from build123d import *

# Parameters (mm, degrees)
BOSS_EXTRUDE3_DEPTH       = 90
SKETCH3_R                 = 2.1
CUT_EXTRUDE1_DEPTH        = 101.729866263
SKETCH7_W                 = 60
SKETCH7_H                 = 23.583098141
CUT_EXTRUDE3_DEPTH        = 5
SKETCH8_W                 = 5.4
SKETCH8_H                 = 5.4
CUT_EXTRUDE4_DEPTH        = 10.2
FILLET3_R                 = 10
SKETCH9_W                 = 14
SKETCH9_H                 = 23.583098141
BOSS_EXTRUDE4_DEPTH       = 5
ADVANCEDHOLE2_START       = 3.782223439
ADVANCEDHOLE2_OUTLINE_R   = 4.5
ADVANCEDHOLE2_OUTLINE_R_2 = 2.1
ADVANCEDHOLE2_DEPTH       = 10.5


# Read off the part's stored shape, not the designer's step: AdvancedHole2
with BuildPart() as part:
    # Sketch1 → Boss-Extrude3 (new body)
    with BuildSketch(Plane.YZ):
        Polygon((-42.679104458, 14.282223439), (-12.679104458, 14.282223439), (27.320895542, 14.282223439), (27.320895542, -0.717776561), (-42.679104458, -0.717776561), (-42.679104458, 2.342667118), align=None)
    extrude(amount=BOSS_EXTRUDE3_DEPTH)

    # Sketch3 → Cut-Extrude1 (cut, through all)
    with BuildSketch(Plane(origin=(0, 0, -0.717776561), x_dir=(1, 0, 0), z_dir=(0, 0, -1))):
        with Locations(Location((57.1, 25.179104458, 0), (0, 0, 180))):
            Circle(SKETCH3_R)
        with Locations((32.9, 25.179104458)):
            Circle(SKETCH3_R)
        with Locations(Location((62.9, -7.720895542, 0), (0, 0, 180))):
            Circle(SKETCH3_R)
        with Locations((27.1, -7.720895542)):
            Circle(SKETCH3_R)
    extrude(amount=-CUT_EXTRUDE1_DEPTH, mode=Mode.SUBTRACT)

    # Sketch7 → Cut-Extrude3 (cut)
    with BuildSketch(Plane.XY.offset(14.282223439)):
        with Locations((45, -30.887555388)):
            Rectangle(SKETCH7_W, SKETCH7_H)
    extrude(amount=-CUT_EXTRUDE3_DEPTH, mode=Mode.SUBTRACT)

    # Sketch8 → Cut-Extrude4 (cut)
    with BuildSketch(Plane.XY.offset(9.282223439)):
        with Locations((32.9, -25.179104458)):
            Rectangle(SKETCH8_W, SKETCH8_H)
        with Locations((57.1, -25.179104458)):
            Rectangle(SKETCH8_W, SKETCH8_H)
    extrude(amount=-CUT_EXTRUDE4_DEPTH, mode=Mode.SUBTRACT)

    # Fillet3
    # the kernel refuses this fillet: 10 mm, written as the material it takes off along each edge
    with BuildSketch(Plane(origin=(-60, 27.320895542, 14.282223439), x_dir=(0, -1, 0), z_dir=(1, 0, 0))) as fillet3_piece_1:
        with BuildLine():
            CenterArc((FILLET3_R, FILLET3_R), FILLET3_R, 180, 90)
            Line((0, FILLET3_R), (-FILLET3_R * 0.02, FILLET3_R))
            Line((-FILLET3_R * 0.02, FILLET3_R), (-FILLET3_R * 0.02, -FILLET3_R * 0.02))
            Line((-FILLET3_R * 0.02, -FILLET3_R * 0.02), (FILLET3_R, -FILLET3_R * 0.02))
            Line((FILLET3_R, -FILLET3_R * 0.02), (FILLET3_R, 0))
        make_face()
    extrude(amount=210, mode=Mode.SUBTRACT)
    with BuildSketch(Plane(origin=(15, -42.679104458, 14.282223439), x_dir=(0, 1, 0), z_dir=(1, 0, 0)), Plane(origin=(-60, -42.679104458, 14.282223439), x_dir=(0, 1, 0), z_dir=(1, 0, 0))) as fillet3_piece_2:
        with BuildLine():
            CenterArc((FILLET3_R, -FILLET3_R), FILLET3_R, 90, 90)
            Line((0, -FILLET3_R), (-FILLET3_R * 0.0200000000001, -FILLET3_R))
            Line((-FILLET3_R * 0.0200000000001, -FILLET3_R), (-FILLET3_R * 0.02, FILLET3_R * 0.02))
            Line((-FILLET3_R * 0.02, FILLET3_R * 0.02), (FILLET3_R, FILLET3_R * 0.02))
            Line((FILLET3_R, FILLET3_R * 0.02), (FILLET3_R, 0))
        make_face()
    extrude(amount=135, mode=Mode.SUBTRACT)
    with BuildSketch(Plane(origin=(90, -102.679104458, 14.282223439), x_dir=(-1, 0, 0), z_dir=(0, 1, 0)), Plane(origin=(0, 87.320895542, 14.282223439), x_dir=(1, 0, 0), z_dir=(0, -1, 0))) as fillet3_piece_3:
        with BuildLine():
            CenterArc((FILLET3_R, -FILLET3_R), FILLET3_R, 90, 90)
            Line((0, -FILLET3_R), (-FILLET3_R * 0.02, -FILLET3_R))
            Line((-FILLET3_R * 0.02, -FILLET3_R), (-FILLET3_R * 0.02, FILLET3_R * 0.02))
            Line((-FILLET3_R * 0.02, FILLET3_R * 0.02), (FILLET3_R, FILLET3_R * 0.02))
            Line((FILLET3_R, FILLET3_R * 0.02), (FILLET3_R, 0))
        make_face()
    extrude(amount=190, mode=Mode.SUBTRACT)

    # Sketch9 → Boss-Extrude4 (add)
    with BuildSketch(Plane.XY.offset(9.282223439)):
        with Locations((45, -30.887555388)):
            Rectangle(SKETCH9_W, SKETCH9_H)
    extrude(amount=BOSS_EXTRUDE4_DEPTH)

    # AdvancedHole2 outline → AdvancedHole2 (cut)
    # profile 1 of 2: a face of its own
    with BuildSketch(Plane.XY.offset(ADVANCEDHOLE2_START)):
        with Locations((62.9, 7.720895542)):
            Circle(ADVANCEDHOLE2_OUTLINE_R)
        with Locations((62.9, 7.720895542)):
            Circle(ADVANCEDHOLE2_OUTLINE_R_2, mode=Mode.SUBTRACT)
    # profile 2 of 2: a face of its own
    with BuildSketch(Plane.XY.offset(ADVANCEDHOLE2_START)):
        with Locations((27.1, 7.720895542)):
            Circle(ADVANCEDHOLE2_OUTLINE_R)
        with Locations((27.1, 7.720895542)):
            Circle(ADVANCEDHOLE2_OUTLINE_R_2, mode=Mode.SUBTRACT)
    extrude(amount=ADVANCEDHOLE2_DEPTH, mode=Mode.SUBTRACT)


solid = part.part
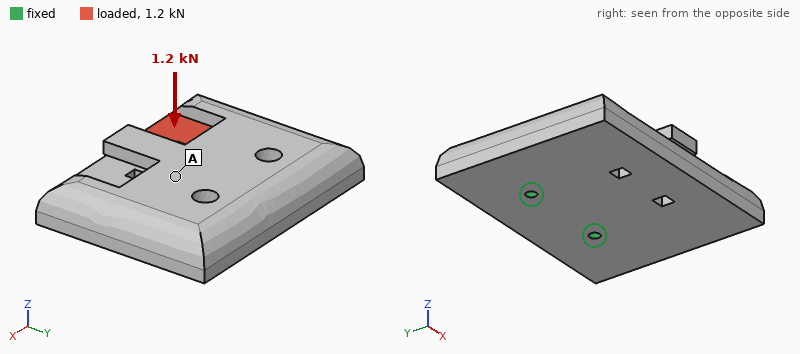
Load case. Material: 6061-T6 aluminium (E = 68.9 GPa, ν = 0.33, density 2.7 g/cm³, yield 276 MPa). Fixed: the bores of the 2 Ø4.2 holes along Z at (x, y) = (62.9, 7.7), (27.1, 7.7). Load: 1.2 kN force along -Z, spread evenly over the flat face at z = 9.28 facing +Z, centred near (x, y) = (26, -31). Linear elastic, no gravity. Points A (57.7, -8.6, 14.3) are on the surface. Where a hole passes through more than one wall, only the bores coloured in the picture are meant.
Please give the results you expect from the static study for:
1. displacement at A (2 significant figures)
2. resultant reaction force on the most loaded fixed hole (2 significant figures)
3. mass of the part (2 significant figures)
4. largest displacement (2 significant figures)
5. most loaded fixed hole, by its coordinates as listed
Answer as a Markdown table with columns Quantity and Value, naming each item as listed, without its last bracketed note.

| Quantity | Value |
|---|---|
| displacement at A | 0.091 mm |
| resultant reaction force on the most loaded fixed hole | 1.2 kN |
| mass of the part | 220 g |
| largest displacement | 0.26 mm |
| most loaded fixed hole, by its coordinates as listed | (27.1, 7.7) |
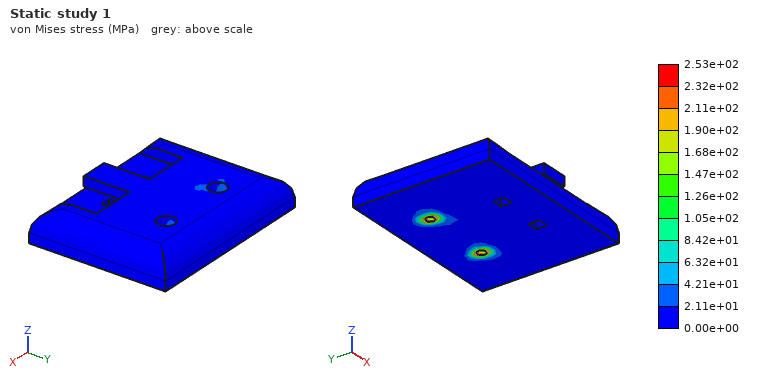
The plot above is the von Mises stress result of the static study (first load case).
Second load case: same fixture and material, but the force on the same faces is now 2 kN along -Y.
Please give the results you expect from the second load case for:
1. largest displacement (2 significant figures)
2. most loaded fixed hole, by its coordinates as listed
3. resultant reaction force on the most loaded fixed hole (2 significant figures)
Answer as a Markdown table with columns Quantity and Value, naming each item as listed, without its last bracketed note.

| Quantity | Value |
|---|---|
| largest displacement | 87 µm |
| most loaded fixed hole, by its coordinates as listed | (27.1, 7.7) |
| resultant reaction force on the most loaded fixed hole | 2.0 kN |
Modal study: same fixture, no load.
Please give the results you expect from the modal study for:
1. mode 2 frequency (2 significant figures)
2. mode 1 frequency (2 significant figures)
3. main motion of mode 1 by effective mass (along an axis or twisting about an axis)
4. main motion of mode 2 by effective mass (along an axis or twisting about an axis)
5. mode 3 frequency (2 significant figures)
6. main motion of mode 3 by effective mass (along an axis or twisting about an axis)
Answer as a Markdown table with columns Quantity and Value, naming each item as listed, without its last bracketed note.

| Quantity | Value |
|---|---|
| mode 2 frequency | 4200 Hz |
| mode 1 frequency | 1400 Hz |
| main motion of mode 1 by effective mass | along Z |
| main motion of mode 2 by effective mass | twisting about Y |
| mode 3 frequency | 5400 Hz |
| main motion of mode 3 by effective mass | along X |
